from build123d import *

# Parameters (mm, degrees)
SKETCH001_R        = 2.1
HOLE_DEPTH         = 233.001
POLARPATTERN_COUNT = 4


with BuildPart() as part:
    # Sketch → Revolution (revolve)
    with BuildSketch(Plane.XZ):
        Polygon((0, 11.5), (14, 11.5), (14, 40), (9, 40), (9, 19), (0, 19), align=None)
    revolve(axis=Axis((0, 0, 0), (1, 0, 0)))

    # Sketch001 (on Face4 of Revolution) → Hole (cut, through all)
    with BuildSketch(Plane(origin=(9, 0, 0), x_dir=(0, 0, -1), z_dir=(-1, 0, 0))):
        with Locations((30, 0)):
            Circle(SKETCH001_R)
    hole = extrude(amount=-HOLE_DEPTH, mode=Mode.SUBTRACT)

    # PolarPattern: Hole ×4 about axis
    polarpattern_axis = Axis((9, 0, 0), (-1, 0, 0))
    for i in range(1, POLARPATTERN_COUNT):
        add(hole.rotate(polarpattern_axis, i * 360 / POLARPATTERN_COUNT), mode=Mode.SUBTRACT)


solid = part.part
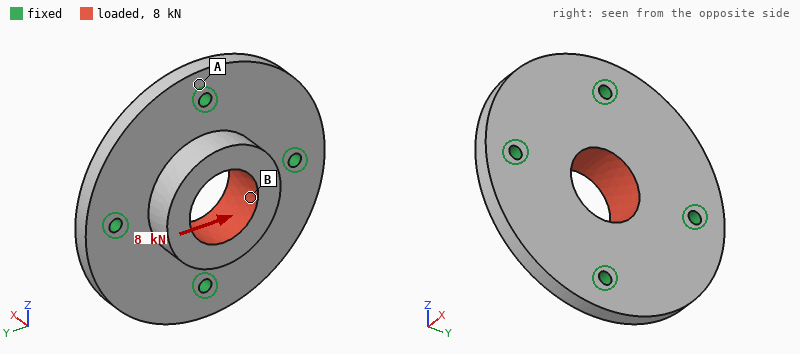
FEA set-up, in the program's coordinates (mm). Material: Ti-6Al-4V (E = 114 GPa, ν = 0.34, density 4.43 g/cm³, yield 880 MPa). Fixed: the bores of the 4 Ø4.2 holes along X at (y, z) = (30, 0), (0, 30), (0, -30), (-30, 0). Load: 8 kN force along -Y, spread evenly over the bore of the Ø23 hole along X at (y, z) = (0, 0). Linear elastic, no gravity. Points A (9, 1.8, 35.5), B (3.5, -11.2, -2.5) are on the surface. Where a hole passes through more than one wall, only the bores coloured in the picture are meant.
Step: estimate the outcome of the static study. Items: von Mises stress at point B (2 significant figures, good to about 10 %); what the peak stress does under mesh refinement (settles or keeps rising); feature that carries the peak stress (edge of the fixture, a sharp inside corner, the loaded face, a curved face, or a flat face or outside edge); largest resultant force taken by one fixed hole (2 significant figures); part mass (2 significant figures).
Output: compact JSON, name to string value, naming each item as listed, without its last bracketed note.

{"von Mises stress at point B": "16 MPa", "what the peak stress does under mesh refinement": "keeps rising", "feature that carries the peak stress": "edge of the fixture", "largest resultant force taken by one fixed hole": "2.5 kN", "part mass": "130 g"}
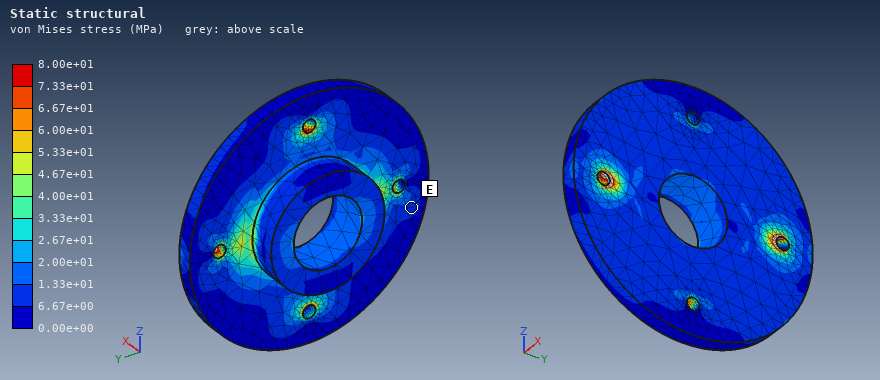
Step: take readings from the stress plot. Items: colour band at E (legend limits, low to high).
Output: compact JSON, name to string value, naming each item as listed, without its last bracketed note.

{"colour band at E": "6.67e+00 to 1.33e+01 MPa"}
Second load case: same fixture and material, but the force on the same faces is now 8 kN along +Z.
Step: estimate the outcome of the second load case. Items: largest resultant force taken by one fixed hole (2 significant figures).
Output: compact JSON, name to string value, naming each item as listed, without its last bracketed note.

{"largest resultant force taken by one fixed hole": "2.5 kN"}
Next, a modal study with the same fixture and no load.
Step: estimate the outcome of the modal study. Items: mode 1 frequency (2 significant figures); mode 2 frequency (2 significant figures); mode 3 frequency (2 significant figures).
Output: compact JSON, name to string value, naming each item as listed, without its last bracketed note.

{"mode 1 frequency": "9300 Hz", "mode 2 frequency": "9800 Hz", "mode 3 frequency": "9800 Hz"}
